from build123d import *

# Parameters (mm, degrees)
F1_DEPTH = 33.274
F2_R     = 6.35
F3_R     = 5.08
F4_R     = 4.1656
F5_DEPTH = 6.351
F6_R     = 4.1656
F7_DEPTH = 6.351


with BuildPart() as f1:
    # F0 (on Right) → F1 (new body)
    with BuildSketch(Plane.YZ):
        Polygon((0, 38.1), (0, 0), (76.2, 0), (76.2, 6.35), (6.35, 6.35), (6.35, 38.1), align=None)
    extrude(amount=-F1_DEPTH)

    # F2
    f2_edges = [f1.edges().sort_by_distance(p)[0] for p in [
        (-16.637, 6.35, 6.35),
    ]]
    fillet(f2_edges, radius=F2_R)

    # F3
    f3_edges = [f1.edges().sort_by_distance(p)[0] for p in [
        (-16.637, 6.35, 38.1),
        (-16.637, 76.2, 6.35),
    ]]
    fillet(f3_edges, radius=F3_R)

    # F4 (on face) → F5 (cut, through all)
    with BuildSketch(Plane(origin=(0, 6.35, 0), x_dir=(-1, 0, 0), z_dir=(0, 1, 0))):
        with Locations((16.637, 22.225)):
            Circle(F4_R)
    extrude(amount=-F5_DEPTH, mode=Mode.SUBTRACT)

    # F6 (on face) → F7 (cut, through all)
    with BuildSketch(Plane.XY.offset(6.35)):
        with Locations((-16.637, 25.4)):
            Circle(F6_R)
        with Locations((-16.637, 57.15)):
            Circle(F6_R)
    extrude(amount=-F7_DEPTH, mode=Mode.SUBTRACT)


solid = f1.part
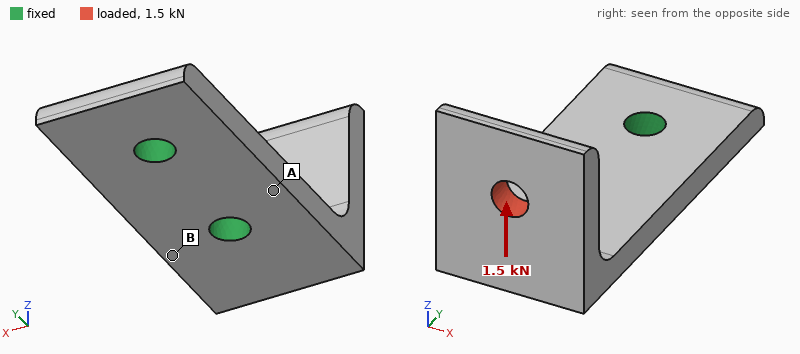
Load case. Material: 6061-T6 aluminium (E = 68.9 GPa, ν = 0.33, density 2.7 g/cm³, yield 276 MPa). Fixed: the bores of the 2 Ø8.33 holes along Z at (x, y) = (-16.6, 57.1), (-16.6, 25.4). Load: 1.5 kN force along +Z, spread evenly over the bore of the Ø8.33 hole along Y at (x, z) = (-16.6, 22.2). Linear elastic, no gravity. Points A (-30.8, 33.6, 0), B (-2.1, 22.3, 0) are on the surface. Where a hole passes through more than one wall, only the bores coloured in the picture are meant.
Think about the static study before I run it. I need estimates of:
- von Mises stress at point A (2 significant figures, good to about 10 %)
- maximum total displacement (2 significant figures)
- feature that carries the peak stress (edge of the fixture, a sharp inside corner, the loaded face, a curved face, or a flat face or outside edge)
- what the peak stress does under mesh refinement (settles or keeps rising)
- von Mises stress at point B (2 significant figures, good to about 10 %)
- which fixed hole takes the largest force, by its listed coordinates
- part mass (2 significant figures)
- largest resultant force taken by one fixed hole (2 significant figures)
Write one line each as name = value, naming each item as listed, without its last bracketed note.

von Mises stress at point A = 17 MPa
maximum total displacement = 0.25 mm
feature that carries the peak stress = edge of the fixture
what the peak stress does under mesh refinement = keeps rising
von Mises stress at point B = 63 MPa
which fixed hole takes the largest force, by its listed coordinates = (-16.6, 25.4)
part mass = 59 g
largest resultant force taken by one fixed hole = 1.7 kN
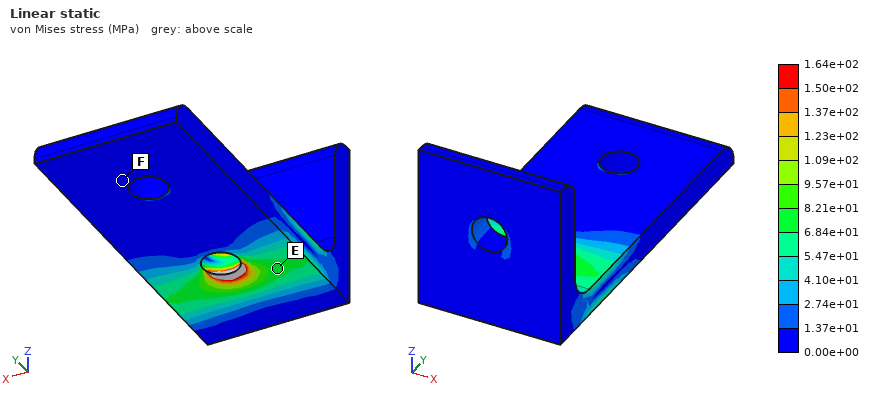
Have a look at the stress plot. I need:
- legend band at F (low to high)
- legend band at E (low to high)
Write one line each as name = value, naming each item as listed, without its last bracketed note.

legend band at F = 0.00e+00 to 1.37e+01 MPa
legend band at E = 6.84e+01 to 8.21e+01 MPa
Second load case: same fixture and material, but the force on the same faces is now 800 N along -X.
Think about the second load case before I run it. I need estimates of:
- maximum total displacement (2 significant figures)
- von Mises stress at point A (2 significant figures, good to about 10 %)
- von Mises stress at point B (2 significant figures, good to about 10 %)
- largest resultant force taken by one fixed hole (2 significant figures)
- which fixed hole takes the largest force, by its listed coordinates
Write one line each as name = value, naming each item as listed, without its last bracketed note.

maximum total displacement = 0.12 mm
von Mises stress at point A = 22 MPa
von Mises stress at point B = 32 MPa
largest resultant force taken by one fixed hole = 1.1 kN
which fixed hole takes the largest force, by its listed coordinates = (-16.6, 25.4)
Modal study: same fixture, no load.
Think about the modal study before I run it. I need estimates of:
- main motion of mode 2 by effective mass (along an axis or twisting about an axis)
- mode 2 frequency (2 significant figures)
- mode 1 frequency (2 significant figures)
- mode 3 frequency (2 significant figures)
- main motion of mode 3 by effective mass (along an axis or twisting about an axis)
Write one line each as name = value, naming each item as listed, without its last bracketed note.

main motion of mode 2 by effective mass = along X
mode 2 frequency = 3500 Hz
mode 1 frequency = 2500 Hz
mode 3 frequency = 7400 Hz
main motion of mode 3 by effective mass = along Z
